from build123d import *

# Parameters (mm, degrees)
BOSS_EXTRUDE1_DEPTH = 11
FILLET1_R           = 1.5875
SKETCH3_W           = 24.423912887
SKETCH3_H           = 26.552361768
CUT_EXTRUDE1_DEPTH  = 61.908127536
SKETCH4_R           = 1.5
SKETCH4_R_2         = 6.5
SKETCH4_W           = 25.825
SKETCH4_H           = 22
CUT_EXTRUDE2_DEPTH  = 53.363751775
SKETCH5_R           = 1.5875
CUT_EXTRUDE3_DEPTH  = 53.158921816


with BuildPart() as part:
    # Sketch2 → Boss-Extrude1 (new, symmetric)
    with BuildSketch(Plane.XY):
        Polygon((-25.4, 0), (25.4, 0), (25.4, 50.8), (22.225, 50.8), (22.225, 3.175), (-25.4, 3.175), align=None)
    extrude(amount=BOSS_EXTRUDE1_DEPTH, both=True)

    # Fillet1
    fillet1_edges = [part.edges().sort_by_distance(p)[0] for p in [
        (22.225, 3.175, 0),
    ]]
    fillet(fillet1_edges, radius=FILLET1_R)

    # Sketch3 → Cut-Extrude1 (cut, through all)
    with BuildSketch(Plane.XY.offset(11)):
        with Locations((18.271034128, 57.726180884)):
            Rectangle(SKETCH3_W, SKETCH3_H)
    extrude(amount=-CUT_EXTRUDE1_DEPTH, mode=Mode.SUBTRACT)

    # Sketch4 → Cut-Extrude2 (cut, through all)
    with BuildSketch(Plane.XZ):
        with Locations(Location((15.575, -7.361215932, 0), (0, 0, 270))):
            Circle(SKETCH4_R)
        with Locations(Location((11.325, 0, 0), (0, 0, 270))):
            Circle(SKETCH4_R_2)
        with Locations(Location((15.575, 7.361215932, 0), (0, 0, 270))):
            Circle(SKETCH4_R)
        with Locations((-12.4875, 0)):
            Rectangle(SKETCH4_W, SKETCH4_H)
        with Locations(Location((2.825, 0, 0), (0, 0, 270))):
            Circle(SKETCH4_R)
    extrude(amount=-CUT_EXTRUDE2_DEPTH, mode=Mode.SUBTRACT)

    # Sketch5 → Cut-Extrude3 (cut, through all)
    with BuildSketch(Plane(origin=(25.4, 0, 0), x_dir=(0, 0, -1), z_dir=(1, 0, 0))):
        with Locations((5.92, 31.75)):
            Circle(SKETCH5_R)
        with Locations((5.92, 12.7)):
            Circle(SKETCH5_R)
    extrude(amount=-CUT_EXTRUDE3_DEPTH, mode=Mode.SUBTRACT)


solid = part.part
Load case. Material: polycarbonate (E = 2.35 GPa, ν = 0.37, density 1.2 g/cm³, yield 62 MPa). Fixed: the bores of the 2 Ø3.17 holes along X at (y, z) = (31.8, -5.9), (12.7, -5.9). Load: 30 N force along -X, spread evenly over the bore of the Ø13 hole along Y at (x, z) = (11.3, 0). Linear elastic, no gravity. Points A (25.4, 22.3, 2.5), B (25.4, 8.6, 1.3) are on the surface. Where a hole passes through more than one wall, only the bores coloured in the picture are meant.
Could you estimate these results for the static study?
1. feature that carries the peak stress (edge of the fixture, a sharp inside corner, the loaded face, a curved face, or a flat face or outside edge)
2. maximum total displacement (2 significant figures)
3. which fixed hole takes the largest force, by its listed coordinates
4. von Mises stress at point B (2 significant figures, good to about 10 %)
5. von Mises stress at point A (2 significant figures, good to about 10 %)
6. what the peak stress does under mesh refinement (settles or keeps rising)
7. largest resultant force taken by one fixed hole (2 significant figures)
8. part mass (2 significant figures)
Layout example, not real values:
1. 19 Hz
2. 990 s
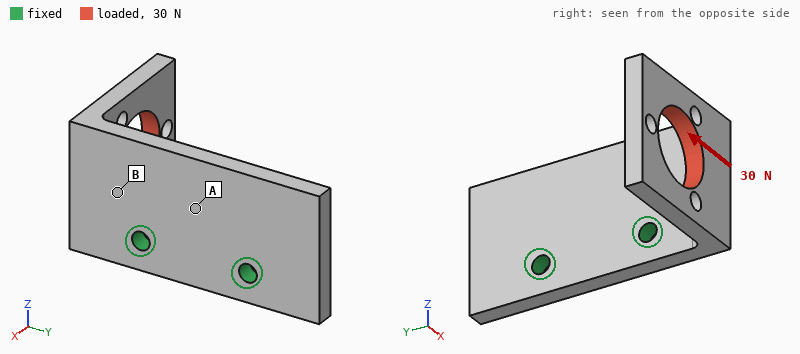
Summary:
1. edge of the fixture
2. 0.50 mm
3. (12.7, -5.9)
4. 4.4 MPa
5. 1.8 MPa
6. keeps rising
7. 36 N
8. 4.9 g
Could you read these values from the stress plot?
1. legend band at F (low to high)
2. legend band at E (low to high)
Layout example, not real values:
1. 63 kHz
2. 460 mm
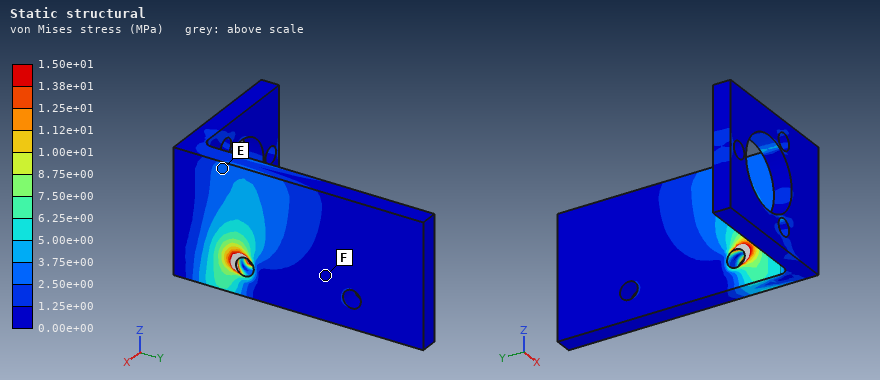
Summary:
1. 0.00e+00 to 1.25e+00 MPa
2. 2.50e+00 to 3.75e+00 MPa
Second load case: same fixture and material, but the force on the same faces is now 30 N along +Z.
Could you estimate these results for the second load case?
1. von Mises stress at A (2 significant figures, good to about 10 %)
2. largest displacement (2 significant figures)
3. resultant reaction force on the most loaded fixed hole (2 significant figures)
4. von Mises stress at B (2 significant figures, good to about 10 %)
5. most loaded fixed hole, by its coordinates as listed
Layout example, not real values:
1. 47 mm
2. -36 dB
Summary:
1. 3.2 MPa
2. 0.64 mm
3. 44 N
4. 3.4 MPa
5. (12.7, -5.9)
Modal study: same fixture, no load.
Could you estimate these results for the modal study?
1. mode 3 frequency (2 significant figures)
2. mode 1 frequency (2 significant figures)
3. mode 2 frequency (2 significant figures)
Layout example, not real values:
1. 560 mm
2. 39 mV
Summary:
1. 2200 Hz
2. 760 Hz
3. 1100 Hz
